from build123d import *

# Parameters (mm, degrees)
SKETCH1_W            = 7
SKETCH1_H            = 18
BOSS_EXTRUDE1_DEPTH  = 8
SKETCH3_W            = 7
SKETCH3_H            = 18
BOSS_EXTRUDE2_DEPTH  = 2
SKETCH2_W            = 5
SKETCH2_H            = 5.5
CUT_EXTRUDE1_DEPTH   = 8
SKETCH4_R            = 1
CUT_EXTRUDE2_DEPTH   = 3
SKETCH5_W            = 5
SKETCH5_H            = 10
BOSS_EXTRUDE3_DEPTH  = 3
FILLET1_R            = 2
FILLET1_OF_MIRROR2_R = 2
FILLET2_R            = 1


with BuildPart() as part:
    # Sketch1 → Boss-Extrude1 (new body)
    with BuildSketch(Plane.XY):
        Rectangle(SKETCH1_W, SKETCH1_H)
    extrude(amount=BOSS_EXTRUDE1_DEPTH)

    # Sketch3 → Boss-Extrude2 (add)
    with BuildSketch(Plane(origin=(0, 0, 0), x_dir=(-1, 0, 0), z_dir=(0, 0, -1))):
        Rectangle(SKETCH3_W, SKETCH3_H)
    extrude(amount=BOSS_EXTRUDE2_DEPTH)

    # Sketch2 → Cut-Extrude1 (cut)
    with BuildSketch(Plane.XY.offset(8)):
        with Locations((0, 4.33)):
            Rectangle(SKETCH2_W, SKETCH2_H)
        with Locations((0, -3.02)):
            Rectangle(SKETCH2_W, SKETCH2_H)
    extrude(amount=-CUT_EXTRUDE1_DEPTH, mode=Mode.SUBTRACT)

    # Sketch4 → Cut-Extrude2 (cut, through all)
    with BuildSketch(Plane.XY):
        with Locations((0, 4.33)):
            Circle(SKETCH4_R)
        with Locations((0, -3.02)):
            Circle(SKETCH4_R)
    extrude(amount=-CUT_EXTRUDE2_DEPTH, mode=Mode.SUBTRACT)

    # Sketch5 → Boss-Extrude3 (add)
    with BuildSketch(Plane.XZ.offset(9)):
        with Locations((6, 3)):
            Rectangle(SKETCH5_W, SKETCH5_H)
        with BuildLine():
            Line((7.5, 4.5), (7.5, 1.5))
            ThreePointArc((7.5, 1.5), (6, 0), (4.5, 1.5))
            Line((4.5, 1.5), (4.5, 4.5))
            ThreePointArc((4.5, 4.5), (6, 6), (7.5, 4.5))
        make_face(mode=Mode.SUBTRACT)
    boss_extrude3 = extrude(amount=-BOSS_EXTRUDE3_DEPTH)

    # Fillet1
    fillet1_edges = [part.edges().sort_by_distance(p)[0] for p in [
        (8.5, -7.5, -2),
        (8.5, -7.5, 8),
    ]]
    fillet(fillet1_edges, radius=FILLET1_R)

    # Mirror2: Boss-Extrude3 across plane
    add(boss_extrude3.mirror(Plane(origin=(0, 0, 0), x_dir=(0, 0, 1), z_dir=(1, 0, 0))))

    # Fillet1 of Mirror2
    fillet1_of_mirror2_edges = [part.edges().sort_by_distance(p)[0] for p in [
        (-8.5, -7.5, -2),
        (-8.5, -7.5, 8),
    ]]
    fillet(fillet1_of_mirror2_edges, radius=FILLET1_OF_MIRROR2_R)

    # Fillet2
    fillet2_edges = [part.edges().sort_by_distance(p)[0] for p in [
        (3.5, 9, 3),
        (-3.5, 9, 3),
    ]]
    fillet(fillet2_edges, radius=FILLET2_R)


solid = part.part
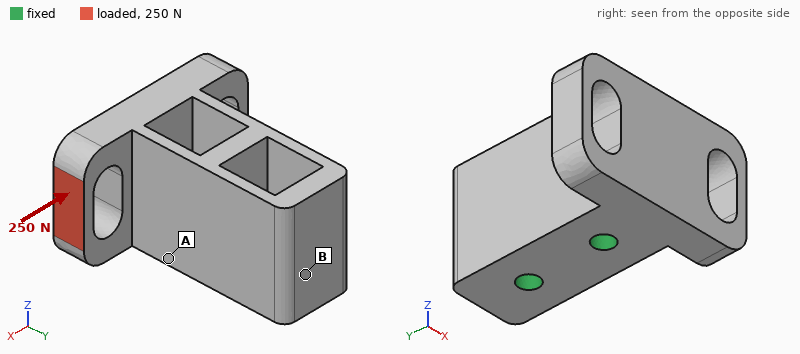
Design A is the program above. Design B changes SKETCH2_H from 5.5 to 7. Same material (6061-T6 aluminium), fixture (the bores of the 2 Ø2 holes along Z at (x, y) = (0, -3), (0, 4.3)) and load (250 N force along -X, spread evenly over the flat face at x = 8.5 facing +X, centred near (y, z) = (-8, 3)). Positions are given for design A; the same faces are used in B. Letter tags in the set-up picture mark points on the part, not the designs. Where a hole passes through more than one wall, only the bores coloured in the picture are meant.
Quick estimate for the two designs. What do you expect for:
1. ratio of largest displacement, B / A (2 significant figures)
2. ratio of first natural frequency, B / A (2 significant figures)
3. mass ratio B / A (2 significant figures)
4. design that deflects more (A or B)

1.2
0.90
0.88
B
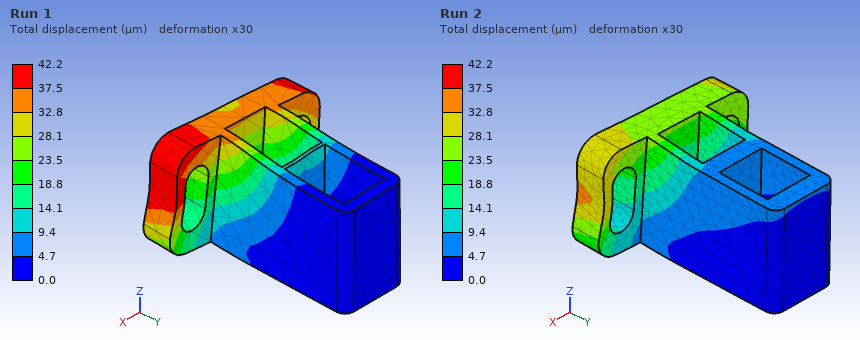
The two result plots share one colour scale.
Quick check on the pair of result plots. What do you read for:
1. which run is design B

Run 1
